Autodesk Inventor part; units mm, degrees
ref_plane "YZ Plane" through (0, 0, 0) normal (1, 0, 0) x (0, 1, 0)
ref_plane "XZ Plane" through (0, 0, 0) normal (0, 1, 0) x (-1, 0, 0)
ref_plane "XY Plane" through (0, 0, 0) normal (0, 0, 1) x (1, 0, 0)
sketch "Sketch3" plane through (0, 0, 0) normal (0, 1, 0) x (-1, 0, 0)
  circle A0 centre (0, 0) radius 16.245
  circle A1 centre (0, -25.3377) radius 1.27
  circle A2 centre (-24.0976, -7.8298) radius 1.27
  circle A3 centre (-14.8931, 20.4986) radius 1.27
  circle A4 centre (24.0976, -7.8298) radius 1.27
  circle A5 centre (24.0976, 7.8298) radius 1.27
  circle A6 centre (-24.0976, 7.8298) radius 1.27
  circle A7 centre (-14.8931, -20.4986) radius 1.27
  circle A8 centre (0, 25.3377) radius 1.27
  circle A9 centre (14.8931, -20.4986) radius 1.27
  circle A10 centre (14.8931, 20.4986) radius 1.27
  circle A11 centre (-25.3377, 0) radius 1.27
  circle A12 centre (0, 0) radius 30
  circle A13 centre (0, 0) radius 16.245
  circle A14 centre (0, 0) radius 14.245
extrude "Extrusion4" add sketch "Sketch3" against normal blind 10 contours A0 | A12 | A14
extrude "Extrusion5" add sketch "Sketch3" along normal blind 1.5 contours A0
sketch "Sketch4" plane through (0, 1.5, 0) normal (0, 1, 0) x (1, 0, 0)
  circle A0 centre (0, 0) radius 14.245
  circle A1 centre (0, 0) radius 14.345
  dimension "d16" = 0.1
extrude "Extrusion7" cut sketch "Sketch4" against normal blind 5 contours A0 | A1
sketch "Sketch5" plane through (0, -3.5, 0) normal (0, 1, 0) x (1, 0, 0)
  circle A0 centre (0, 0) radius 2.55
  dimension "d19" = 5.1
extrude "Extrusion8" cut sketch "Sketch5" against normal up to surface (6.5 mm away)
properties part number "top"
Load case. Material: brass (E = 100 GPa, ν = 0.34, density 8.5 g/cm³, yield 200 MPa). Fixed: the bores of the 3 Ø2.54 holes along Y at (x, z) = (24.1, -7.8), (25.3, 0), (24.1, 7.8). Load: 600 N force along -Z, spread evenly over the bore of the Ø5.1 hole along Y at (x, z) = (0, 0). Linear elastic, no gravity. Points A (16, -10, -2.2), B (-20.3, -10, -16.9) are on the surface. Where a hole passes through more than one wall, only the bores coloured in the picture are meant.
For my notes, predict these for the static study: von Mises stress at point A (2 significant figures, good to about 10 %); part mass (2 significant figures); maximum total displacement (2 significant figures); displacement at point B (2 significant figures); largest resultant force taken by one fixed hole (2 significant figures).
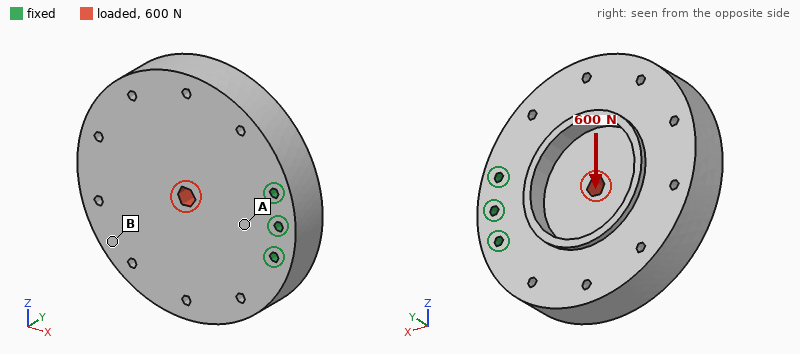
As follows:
7.8 MPa
220 g
8.1 µm
7.2 µm
850 N
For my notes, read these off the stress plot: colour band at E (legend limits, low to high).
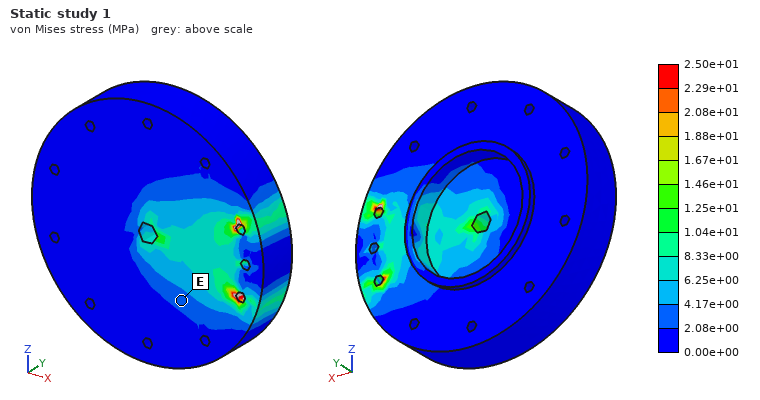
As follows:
2.08e+00 to 4.17e+00 MPa
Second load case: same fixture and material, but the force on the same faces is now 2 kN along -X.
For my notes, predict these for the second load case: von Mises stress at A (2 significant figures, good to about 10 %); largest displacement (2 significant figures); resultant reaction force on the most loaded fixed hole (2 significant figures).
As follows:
13 MPa
8.9 µm
790 N
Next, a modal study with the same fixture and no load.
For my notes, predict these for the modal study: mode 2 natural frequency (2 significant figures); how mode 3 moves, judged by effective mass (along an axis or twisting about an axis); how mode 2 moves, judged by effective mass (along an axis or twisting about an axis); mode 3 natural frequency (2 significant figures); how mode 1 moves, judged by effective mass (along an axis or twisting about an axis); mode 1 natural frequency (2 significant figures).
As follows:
3200 Hz
along Z
along Z
3500 Hz
along Y
1600 Hz
